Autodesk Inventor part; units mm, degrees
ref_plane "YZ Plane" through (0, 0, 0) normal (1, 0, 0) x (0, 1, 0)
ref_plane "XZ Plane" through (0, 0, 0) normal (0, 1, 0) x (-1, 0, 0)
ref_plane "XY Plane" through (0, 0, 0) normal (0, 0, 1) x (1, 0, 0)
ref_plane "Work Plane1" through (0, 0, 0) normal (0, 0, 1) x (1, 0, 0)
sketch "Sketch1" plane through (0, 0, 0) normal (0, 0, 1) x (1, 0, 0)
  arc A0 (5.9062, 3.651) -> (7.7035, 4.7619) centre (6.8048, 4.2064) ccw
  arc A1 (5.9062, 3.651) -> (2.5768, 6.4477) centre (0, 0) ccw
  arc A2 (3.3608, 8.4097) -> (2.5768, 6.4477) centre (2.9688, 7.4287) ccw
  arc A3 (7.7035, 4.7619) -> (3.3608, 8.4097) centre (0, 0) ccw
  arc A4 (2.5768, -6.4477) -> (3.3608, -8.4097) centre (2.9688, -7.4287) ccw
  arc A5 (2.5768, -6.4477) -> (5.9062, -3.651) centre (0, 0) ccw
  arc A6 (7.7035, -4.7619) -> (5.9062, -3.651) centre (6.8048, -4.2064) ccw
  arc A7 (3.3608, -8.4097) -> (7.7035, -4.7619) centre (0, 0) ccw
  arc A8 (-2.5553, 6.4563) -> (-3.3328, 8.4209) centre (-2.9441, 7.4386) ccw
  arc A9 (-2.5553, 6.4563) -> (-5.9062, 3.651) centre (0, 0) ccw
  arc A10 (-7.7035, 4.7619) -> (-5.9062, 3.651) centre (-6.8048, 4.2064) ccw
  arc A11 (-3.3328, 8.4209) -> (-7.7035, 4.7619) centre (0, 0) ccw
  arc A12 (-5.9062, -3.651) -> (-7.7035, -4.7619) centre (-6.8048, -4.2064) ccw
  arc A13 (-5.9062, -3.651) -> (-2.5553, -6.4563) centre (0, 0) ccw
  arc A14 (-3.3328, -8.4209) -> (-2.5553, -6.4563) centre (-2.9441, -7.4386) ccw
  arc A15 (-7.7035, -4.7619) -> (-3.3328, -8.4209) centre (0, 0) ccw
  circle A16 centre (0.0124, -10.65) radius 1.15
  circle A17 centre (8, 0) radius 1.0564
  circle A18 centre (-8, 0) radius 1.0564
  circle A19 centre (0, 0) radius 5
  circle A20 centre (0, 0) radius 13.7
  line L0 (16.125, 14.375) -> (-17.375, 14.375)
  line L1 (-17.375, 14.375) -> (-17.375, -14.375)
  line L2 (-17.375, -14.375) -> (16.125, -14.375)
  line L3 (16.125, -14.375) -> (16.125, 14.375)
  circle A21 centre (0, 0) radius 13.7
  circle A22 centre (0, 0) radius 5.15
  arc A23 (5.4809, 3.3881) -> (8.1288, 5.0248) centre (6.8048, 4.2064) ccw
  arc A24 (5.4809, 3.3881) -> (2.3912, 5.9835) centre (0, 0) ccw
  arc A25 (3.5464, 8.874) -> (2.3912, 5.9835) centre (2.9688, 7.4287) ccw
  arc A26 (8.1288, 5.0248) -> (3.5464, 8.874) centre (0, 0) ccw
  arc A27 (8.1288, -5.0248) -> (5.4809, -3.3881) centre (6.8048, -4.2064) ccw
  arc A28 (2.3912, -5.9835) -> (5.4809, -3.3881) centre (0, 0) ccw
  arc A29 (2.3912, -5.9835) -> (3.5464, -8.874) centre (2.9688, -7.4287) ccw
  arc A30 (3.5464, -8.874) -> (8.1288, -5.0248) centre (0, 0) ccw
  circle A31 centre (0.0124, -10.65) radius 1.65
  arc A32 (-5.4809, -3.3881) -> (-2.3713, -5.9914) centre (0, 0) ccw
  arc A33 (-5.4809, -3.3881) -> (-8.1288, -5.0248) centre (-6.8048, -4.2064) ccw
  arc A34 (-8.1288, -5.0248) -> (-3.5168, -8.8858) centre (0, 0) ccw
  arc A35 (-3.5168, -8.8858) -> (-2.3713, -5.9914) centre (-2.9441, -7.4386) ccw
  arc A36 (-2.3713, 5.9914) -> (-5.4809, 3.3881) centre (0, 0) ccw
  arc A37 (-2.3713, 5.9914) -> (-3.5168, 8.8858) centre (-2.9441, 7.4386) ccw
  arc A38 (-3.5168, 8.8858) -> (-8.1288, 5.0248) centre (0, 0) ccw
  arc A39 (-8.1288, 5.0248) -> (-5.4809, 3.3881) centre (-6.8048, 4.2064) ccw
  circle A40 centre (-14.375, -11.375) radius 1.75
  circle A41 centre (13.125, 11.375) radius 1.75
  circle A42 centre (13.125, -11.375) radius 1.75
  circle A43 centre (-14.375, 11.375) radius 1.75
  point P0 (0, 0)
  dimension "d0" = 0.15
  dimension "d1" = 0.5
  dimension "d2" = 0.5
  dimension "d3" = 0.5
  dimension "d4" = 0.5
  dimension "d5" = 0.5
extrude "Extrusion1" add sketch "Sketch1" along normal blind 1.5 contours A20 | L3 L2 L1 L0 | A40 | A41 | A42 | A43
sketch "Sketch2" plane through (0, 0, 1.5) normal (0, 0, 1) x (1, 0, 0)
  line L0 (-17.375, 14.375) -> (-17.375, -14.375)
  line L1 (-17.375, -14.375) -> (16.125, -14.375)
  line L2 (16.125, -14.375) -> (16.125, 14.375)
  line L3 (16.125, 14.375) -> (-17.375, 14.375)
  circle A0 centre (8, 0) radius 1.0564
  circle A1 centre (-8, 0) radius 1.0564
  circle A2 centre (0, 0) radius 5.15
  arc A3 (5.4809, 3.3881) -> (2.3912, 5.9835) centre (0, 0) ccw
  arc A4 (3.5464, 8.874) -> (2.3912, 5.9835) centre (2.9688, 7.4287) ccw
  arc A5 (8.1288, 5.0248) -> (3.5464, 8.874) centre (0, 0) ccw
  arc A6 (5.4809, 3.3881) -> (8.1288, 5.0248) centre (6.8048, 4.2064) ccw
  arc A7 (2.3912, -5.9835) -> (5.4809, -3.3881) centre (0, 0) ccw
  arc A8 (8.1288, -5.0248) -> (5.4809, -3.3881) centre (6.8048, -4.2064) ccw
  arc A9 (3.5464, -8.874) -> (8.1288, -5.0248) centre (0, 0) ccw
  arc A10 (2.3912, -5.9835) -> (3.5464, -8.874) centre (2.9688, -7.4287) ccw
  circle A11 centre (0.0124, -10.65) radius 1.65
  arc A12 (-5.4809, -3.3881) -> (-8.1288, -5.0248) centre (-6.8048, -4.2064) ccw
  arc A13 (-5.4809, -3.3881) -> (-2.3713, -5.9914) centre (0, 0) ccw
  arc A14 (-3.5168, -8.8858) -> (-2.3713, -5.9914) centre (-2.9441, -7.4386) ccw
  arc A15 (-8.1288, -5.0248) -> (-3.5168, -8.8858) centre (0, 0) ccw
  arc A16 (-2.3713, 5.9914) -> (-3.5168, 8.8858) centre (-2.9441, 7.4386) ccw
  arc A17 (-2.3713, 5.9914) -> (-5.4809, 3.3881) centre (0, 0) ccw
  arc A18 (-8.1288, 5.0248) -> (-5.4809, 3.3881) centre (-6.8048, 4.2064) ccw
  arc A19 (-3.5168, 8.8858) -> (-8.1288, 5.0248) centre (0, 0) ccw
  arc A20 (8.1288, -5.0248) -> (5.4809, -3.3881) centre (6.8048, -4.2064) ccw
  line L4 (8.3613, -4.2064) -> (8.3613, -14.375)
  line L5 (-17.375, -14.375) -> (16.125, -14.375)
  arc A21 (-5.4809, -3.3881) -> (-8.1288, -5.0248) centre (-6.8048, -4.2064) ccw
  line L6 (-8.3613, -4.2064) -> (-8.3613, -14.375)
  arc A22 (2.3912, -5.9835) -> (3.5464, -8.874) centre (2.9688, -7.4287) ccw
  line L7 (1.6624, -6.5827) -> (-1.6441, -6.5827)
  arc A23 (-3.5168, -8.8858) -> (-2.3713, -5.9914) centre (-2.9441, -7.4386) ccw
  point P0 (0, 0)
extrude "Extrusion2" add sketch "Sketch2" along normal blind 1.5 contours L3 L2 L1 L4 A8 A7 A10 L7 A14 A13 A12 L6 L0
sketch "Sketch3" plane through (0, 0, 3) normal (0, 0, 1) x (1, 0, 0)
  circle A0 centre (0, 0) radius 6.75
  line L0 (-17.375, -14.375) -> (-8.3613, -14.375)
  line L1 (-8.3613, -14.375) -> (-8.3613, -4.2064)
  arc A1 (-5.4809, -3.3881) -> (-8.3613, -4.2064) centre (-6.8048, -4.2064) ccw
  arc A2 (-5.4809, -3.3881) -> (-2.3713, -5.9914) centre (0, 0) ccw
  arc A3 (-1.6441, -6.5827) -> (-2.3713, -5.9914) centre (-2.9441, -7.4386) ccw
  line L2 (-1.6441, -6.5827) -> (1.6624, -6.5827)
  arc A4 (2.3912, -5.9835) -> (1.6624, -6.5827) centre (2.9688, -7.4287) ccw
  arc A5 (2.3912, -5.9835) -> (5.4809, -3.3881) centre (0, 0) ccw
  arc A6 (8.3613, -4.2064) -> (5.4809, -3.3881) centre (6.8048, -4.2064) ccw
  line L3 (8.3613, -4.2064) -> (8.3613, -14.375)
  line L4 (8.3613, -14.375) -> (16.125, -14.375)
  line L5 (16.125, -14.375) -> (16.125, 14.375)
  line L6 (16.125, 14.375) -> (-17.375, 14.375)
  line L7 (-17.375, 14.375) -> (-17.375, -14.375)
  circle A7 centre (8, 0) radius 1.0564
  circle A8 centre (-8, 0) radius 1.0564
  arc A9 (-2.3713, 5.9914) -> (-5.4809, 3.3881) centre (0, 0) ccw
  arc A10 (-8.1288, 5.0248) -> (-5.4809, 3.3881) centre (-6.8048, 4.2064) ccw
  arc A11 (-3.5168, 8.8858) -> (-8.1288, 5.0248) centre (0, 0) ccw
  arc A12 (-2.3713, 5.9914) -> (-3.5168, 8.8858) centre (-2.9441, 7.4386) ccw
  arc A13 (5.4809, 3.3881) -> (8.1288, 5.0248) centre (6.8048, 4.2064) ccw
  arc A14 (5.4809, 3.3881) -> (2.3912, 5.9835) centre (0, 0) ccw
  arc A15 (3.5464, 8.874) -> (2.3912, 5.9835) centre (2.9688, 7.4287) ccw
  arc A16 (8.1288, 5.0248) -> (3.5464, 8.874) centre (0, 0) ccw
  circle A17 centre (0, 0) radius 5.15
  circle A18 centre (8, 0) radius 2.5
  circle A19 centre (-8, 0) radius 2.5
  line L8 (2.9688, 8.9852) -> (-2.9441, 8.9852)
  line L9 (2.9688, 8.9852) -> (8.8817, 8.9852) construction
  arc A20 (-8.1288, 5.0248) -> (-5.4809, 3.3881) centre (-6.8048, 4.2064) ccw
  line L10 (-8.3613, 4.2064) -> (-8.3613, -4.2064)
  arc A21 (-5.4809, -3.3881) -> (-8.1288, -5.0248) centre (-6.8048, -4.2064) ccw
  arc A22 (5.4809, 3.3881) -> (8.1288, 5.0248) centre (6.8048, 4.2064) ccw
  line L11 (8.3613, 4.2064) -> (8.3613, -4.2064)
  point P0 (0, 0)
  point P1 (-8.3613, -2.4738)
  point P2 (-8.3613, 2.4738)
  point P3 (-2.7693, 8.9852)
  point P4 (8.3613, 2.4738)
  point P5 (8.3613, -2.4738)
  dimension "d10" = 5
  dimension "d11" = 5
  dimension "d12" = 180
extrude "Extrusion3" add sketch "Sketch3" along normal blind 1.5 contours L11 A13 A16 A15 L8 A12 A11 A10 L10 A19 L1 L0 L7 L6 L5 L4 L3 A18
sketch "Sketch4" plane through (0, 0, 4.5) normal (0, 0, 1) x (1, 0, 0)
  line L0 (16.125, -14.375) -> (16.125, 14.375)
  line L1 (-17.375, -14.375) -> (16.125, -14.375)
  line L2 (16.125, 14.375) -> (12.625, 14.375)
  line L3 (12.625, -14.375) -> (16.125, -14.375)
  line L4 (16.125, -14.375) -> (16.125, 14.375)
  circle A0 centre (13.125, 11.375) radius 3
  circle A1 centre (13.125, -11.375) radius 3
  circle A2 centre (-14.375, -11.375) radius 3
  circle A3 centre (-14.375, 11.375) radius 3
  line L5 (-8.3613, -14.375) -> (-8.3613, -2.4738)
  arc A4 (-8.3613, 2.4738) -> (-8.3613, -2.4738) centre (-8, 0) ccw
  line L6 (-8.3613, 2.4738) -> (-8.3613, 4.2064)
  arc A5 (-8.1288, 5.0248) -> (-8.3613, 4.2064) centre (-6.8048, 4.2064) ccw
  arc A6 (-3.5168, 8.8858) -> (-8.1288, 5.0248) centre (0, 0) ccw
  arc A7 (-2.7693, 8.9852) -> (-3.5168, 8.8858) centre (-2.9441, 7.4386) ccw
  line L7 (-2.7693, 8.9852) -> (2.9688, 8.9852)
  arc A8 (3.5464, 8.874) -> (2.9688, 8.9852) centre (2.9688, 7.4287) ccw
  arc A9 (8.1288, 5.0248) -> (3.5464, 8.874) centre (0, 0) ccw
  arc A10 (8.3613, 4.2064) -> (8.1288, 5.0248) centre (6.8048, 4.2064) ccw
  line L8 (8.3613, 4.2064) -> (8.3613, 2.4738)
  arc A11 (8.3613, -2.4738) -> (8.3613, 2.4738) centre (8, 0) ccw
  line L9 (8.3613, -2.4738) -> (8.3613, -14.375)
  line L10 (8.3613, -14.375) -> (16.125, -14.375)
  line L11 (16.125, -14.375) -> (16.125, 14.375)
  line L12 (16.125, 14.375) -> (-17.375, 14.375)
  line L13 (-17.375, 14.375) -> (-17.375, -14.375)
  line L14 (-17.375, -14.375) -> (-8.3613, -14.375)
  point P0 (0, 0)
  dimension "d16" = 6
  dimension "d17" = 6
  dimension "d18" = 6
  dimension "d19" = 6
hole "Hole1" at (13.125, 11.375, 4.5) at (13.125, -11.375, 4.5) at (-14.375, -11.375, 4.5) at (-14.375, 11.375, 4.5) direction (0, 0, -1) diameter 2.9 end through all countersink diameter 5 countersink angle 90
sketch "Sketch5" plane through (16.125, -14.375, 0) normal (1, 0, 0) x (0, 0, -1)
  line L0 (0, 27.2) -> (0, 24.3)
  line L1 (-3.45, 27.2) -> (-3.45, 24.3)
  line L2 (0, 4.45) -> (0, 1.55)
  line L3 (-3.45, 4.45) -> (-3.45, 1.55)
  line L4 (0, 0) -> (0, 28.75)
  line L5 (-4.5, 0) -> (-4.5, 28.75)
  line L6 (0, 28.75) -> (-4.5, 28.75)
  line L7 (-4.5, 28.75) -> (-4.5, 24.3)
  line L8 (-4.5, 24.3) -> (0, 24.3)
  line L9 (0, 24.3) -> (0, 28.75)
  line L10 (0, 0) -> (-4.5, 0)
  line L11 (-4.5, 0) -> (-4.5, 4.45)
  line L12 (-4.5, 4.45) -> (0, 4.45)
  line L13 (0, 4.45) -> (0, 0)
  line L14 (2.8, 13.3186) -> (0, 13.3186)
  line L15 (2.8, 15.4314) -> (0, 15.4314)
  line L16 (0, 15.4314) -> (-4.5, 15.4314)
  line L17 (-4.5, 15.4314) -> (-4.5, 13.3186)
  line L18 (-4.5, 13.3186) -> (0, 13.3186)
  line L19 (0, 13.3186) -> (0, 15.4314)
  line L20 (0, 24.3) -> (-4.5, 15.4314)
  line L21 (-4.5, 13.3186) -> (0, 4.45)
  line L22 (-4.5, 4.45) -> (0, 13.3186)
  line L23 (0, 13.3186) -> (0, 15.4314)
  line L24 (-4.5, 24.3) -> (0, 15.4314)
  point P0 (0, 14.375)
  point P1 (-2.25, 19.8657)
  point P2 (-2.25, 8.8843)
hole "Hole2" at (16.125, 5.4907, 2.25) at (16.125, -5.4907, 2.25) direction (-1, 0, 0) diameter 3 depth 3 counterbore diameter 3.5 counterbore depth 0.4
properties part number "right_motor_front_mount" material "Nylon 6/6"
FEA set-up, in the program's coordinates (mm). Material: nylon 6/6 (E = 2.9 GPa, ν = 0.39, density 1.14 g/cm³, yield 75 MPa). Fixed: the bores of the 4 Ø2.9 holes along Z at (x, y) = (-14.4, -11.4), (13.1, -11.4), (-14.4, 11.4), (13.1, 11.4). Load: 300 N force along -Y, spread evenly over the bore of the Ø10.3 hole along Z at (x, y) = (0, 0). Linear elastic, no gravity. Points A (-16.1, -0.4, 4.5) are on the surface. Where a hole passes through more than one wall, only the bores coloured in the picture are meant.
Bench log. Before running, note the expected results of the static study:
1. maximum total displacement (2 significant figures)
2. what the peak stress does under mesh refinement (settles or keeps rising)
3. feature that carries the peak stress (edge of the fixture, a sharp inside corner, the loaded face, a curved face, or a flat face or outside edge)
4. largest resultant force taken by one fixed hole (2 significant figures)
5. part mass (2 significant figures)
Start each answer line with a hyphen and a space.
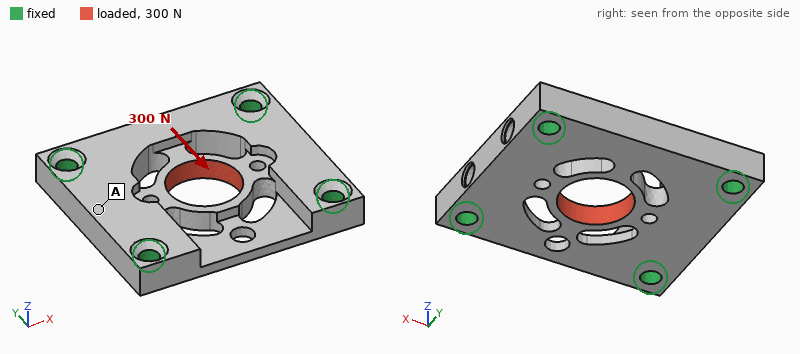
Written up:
- 81 µm
- keeps rising
- a sharp inside corner
- 89 N
- 3.2 g
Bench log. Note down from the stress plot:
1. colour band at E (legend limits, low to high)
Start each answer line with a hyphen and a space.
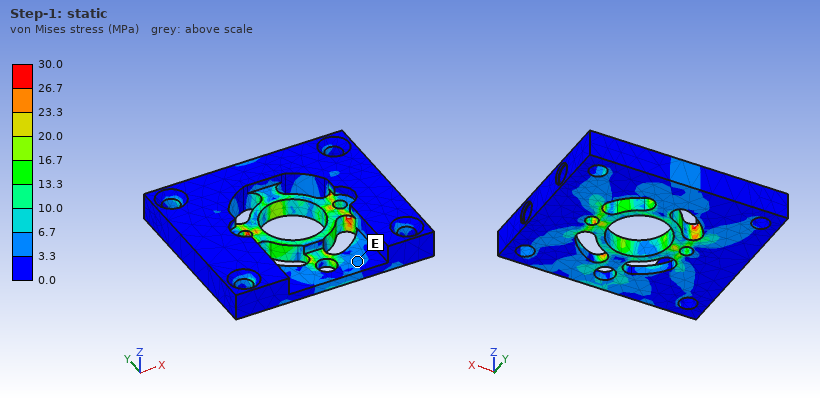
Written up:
- 3.3 to 6.7 MPa
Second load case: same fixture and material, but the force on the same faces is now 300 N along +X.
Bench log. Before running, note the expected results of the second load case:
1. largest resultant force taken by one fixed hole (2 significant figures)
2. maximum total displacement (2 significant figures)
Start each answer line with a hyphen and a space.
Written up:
- 93 N
- 0.12 mm
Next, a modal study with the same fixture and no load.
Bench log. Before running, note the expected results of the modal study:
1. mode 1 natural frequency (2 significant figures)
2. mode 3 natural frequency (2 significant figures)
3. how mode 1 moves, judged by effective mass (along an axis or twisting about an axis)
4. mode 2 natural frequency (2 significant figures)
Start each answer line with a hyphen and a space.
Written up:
- 6700 Hz
- 9800 Hz
- along Z
- 8100 Hz
